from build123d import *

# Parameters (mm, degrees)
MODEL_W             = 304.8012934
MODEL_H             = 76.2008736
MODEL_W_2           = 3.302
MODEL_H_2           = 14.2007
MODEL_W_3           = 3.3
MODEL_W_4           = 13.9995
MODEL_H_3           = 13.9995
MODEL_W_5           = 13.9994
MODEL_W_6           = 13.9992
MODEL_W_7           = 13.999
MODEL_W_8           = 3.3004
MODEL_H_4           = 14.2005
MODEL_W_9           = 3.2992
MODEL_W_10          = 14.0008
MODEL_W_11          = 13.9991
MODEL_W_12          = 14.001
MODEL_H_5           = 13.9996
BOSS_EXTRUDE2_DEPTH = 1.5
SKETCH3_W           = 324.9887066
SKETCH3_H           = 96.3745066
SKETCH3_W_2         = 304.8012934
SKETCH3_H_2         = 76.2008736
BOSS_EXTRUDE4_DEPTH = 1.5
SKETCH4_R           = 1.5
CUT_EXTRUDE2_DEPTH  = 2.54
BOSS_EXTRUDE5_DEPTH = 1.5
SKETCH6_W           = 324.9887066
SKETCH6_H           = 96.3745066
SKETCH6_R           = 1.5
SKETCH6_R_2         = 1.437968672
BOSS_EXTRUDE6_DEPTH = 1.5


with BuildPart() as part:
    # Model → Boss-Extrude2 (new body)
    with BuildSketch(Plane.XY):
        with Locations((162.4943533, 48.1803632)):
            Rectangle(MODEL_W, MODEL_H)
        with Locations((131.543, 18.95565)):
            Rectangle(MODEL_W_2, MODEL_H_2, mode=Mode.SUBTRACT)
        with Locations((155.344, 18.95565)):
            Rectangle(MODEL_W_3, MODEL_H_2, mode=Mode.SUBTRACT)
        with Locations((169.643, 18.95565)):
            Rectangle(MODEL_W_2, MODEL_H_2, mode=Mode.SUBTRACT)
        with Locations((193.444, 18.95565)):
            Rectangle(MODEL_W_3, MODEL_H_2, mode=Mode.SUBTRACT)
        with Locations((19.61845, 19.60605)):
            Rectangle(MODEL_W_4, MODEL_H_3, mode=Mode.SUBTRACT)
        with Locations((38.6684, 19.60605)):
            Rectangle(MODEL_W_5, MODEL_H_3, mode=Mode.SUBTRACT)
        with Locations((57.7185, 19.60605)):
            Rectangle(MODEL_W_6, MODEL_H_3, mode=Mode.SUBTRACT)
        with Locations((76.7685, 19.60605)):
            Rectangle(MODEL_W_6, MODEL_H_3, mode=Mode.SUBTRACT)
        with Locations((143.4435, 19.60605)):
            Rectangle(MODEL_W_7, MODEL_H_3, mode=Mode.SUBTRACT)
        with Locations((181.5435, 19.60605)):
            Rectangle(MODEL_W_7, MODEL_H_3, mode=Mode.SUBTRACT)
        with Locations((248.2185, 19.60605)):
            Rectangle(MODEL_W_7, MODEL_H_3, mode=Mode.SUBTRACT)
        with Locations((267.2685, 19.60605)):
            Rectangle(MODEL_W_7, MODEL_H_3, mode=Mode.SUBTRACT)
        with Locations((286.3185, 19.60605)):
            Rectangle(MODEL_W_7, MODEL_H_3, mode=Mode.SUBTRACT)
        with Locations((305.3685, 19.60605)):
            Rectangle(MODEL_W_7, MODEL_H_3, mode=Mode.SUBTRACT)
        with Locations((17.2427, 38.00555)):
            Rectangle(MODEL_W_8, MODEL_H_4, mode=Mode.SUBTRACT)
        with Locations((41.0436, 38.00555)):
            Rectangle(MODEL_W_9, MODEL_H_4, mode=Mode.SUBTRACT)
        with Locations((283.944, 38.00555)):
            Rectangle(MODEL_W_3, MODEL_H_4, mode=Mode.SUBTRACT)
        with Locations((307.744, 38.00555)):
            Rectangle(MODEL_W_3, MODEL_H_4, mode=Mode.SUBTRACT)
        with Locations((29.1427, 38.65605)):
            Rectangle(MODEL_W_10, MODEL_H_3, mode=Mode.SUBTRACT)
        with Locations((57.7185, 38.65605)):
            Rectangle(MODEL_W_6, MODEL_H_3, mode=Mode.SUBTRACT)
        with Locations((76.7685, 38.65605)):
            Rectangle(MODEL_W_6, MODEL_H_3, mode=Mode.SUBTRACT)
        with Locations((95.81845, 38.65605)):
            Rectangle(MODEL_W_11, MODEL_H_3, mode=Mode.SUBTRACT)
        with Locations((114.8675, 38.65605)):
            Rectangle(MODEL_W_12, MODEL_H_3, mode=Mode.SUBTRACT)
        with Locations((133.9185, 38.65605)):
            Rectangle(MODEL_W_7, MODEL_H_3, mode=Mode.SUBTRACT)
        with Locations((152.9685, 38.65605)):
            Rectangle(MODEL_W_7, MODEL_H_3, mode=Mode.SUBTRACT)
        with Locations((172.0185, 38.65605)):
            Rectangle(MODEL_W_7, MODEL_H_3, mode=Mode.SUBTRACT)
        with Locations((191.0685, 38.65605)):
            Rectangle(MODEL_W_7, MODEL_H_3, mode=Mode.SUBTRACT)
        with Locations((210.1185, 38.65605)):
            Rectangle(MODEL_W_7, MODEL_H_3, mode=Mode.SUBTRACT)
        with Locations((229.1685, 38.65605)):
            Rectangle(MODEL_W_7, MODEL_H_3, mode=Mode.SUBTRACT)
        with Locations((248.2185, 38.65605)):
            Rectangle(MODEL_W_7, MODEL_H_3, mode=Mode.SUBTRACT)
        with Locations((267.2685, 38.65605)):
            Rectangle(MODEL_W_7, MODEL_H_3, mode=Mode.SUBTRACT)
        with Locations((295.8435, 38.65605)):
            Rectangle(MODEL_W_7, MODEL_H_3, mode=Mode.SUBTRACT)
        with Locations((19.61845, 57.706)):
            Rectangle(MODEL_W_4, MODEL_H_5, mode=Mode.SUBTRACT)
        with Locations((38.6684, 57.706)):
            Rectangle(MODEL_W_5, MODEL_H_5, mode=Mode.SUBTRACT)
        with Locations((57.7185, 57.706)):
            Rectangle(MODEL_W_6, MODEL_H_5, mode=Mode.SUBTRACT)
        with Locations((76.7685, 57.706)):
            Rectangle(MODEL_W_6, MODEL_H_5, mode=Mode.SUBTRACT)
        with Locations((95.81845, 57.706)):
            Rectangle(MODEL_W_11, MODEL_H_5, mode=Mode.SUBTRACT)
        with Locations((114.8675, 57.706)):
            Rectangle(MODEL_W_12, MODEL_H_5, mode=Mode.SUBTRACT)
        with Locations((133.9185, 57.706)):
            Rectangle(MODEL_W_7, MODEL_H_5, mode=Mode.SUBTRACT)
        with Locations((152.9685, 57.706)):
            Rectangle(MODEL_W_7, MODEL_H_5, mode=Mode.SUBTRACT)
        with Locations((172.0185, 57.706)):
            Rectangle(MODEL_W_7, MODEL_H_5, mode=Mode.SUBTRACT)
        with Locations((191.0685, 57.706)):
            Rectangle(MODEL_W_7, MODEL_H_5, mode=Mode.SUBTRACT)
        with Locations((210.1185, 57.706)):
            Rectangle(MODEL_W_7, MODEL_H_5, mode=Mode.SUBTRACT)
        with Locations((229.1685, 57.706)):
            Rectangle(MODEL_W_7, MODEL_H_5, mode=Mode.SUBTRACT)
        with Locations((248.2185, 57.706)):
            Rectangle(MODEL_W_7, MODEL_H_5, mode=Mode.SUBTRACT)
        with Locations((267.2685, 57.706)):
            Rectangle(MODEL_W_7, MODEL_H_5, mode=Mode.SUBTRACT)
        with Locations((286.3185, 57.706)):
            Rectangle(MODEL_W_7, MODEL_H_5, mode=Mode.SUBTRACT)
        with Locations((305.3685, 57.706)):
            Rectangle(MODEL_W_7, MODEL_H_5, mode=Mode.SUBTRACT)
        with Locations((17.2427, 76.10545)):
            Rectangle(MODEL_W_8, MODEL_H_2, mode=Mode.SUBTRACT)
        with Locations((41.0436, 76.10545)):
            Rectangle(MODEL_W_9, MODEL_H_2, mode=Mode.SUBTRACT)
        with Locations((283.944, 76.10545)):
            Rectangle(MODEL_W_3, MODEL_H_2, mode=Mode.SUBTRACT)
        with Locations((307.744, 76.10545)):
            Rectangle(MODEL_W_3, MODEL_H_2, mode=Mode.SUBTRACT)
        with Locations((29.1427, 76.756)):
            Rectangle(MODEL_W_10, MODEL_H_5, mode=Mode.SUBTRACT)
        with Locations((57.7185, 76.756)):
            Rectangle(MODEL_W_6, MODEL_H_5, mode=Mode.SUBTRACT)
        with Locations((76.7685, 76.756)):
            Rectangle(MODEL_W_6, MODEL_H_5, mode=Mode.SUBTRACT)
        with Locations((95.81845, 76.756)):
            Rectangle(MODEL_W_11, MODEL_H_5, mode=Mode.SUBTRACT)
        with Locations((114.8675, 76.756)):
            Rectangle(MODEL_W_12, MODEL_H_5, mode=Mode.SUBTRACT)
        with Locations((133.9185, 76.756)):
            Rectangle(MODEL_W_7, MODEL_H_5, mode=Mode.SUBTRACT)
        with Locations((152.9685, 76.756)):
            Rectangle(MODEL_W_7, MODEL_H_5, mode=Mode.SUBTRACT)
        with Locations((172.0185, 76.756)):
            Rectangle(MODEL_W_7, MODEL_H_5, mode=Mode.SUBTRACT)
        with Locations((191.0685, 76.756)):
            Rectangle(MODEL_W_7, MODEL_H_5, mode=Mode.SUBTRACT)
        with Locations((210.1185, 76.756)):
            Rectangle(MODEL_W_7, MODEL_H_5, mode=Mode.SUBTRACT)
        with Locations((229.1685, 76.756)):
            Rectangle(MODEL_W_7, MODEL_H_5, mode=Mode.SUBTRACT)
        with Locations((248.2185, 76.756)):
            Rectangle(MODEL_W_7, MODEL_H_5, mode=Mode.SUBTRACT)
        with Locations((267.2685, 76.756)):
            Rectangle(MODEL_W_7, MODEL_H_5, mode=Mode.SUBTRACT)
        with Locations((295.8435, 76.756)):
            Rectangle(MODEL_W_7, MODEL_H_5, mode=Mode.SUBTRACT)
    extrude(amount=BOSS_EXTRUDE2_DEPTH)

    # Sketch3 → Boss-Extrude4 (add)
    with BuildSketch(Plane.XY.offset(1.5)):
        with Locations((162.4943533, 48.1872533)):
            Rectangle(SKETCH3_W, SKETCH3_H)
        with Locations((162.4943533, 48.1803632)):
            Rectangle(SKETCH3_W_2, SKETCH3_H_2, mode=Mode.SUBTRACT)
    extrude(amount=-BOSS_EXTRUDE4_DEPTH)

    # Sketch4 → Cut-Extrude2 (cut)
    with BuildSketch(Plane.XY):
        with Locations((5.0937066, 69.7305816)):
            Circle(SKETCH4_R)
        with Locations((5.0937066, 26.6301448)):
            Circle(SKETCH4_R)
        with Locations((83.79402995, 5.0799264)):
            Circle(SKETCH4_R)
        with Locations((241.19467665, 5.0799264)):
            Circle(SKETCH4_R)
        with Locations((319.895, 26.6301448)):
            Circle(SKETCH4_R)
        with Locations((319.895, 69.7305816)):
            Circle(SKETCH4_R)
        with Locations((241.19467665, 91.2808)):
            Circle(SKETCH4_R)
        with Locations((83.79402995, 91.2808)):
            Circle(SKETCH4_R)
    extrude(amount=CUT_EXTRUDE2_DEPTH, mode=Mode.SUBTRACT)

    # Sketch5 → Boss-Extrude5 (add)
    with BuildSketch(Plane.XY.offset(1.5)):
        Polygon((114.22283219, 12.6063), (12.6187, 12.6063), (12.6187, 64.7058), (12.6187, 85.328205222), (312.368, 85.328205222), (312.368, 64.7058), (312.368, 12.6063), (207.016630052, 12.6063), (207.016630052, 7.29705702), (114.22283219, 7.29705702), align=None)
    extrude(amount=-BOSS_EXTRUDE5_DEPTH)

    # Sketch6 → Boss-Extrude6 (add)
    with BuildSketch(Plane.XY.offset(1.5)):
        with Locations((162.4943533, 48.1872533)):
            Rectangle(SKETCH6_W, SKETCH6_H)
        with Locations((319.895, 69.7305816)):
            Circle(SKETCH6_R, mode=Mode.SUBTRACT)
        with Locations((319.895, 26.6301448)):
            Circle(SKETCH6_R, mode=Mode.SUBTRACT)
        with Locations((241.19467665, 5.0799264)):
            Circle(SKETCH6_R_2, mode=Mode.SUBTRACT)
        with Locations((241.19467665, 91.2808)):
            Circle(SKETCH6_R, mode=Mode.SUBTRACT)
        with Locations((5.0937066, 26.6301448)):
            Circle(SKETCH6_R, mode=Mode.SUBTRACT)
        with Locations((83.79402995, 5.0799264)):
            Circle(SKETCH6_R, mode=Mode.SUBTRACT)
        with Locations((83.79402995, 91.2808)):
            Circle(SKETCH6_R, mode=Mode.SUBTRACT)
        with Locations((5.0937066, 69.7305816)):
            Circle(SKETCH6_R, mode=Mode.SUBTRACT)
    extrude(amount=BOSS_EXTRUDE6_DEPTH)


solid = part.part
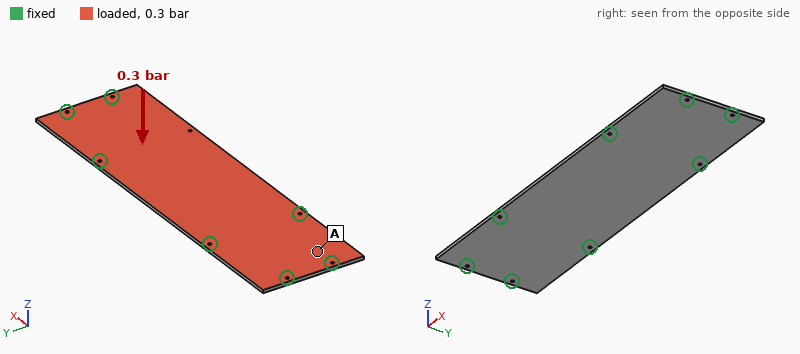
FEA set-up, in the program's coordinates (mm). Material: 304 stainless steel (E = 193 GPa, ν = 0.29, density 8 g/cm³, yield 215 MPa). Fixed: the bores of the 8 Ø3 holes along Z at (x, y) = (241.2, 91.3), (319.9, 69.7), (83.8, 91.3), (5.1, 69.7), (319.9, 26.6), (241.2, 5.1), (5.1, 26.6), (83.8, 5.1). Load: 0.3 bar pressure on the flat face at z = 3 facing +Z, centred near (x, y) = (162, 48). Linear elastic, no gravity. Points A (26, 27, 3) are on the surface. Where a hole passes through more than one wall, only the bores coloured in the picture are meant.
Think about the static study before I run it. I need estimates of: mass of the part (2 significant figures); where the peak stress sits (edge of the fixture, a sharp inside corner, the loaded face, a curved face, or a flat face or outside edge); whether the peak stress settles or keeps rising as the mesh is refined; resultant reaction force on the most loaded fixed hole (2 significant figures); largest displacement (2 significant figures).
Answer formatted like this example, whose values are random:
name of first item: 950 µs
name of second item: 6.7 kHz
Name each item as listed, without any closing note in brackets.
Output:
mass of the part: 750 g
where the peak stress sits: edge of the fixture
whether the peak stress settles or keeps rising as the mesh is refined: keeps rising
resultant reaction force on the most loaded fixed hole: 210 N
largest displacement: 0.15 mm
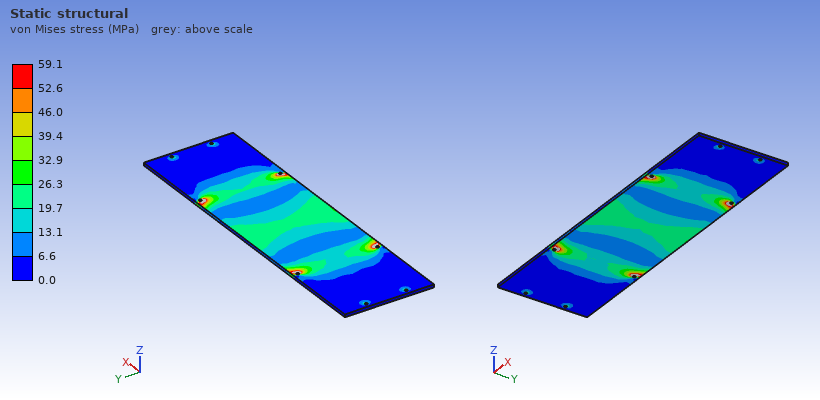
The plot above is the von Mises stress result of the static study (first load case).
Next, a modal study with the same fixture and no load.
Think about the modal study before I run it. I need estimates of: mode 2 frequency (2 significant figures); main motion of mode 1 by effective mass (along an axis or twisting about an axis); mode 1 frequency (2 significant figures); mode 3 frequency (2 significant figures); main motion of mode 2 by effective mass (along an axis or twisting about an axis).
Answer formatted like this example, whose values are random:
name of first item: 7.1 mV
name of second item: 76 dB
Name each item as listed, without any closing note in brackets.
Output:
mode 2 frequency: 880 Hz
main motion of mode 1 by effective mass: along Z
mode 1 frequency: 510 Hz
mode 3 frequency: 1300 Hz
main motion of mode 2 by effective mass: twisting about X
